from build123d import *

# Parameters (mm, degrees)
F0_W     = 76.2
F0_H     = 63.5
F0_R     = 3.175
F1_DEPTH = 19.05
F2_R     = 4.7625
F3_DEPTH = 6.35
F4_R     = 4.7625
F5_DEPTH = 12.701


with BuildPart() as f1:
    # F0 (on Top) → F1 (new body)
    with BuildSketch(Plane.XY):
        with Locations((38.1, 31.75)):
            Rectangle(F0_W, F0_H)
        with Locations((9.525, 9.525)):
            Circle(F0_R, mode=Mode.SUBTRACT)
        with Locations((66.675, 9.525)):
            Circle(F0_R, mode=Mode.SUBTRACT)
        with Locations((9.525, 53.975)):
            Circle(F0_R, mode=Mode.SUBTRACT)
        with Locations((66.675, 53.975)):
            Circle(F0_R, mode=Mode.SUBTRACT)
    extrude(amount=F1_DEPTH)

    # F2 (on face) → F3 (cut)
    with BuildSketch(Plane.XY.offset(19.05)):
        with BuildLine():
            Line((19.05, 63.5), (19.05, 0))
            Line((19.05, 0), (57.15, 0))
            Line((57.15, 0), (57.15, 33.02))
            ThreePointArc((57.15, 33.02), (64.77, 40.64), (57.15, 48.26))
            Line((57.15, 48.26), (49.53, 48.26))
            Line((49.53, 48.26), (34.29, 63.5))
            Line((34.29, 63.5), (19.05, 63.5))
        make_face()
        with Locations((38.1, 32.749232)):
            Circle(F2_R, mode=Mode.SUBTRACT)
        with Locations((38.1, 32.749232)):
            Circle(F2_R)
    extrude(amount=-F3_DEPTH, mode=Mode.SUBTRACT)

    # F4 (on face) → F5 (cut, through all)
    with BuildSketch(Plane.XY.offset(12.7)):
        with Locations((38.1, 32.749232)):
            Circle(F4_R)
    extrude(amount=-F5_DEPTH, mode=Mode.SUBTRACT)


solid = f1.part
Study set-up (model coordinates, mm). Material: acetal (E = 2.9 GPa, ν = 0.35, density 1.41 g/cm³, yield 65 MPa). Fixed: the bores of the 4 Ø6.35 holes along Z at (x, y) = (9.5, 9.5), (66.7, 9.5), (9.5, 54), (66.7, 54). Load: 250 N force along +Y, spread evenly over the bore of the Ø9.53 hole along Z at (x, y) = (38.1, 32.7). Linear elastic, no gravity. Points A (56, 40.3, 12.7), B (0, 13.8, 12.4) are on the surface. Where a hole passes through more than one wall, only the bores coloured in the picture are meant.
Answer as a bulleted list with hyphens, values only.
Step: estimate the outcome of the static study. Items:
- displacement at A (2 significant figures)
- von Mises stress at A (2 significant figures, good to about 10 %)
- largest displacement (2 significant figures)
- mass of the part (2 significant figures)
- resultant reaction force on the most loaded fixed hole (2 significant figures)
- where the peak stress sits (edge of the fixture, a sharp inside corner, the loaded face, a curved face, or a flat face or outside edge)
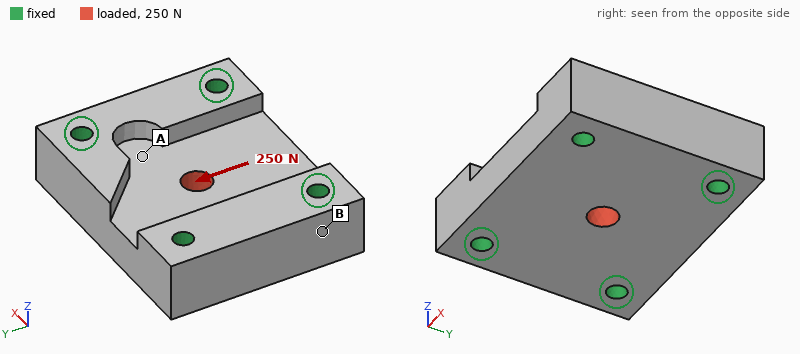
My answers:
- 1.7 µm
- 0.32 MPa
- 5.7 µm
- 100 g
- 74 N
- the loaded face
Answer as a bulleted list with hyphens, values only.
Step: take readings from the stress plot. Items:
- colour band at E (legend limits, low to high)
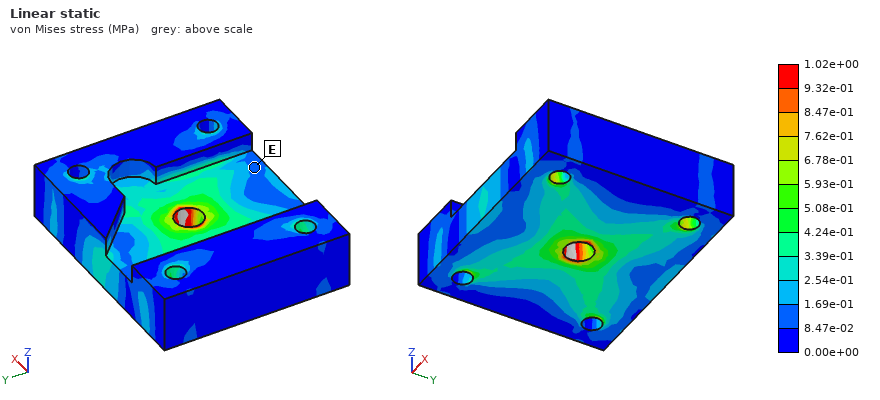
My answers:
- 8.47e-02 to 1.69e-01 MPa
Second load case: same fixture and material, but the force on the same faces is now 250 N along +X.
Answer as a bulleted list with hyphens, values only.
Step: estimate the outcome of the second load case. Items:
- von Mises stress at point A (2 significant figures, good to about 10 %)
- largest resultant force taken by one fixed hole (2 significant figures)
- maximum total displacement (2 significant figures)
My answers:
- 0.31 MPa
- 71 N
- 4.4 µm
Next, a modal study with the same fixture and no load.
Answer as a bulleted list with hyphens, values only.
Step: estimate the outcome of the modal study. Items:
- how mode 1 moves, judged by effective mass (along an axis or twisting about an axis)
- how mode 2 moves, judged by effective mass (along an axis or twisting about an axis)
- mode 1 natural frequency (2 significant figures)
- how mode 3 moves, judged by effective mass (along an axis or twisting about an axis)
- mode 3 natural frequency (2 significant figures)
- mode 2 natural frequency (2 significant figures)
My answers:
- along Z
- twisting about X
- 4700 Hz
- along Y
- 6900 Hz
- 5900 Hz
